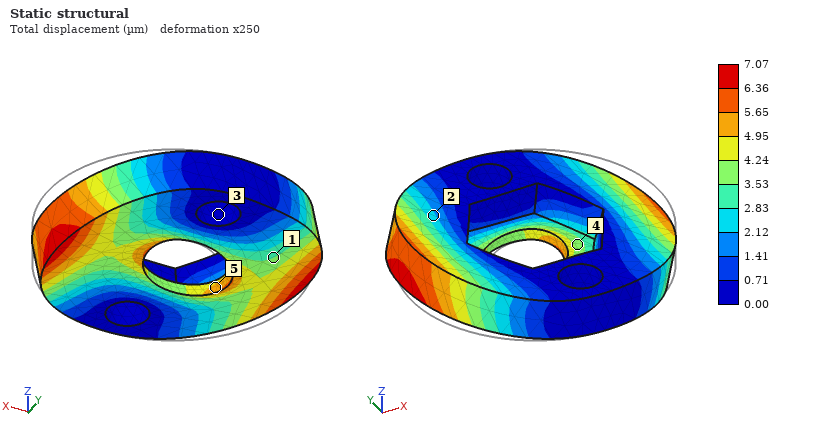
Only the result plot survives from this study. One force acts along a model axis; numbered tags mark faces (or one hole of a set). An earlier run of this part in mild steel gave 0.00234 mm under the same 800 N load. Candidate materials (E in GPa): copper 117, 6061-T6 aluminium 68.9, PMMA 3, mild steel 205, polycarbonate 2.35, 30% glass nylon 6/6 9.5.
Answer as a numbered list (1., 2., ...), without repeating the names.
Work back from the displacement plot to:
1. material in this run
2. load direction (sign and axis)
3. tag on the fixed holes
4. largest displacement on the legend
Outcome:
1. 6061-T6 aluminium
2. -X
3. 3
4. 7.07 µm
